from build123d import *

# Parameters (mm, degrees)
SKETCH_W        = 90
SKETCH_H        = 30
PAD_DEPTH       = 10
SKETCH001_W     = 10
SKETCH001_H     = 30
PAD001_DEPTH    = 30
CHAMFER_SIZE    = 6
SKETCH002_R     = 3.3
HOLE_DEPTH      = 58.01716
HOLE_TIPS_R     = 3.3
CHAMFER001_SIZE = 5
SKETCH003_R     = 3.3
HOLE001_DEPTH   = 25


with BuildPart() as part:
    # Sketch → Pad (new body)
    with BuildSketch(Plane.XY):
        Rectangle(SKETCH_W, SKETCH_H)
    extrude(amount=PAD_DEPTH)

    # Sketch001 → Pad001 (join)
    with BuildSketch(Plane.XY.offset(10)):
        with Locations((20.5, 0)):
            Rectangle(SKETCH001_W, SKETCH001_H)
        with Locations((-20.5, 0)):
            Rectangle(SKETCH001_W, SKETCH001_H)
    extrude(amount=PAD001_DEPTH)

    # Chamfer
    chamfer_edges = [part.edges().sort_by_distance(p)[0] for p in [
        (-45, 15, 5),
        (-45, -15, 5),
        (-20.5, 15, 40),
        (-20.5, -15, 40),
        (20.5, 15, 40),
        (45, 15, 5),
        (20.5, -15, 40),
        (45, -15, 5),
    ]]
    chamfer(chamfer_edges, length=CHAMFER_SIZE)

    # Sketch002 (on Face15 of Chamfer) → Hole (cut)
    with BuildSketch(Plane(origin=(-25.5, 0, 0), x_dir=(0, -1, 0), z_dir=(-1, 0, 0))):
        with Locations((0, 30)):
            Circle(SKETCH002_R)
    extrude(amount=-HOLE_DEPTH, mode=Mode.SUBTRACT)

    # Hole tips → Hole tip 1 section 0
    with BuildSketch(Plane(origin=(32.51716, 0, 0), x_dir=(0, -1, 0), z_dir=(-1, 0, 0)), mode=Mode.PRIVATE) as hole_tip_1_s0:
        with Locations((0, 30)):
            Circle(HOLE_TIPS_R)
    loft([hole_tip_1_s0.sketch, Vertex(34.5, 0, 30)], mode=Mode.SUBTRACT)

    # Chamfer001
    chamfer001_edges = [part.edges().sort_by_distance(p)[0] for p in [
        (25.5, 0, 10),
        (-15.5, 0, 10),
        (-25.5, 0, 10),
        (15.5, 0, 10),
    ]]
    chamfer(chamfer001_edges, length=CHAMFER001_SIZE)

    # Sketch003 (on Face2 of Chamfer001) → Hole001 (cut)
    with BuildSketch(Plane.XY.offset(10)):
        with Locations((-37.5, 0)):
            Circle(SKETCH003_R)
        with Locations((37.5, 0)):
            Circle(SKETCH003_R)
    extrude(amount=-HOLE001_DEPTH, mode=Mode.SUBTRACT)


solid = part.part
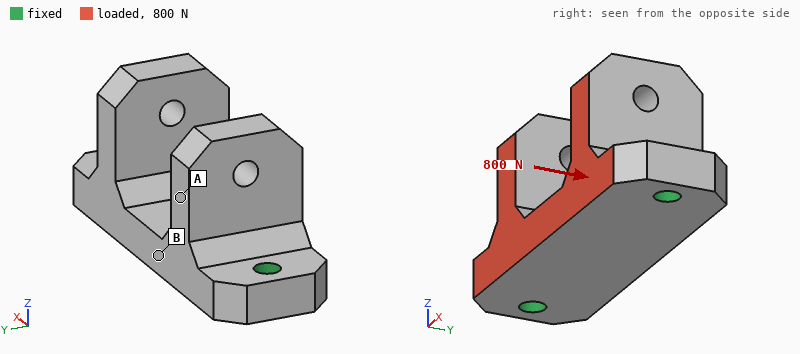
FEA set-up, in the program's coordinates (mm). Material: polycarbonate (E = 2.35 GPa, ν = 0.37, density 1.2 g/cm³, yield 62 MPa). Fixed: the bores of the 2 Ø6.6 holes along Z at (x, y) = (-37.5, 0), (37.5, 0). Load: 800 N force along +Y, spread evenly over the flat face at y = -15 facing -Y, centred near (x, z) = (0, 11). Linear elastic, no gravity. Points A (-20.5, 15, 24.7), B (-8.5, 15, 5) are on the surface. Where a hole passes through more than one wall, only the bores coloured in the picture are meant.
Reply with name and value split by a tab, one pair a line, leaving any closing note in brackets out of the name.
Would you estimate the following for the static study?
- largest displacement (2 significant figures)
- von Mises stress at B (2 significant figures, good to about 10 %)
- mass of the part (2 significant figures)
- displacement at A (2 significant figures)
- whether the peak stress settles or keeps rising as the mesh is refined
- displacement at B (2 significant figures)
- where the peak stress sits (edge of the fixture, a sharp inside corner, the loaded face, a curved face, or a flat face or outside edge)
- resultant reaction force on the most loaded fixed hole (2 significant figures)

largest displacement	0.21 mm
von Mises stress at B	2.7 MPa
mass of the part	52 g
displacement at A	0.15 mm
whether the peak stress settles or keeps rising as the mesh is refined	keeps rising
displacement at B	0.084 mm
where the peak stress sits	edge of the fixture
resultant reaction force on the most loaded fixed hole	400 N
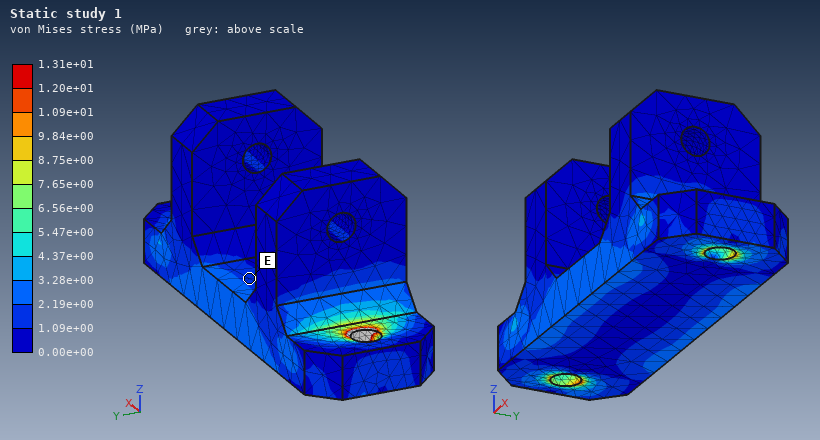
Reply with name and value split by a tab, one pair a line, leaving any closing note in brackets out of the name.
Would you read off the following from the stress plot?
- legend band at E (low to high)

legend band at E	1.09e+00 to 2.19e+00 MPa
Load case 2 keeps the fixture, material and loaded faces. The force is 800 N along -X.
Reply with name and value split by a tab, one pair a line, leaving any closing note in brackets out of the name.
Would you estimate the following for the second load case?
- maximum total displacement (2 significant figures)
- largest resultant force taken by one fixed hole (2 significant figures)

maximum total displacement	0.11 mm
largest resultant force taken by one fixed hole	430 N
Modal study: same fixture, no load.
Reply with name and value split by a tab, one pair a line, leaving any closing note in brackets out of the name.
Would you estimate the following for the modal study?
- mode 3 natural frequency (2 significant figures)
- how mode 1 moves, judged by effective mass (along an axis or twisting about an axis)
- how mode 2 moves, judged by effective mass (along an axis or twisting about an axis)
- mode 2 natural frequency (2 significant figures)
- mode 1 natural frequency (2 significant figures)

mode 3 natural frequency	2100 Hz
how mode 1 moves, judged by effective mass	along Z
how mode 2 moves, judged by effective mass	along Y
mode 2 natural frequency	1500 Hz
mode 1 natural frequency	1400 Hz
